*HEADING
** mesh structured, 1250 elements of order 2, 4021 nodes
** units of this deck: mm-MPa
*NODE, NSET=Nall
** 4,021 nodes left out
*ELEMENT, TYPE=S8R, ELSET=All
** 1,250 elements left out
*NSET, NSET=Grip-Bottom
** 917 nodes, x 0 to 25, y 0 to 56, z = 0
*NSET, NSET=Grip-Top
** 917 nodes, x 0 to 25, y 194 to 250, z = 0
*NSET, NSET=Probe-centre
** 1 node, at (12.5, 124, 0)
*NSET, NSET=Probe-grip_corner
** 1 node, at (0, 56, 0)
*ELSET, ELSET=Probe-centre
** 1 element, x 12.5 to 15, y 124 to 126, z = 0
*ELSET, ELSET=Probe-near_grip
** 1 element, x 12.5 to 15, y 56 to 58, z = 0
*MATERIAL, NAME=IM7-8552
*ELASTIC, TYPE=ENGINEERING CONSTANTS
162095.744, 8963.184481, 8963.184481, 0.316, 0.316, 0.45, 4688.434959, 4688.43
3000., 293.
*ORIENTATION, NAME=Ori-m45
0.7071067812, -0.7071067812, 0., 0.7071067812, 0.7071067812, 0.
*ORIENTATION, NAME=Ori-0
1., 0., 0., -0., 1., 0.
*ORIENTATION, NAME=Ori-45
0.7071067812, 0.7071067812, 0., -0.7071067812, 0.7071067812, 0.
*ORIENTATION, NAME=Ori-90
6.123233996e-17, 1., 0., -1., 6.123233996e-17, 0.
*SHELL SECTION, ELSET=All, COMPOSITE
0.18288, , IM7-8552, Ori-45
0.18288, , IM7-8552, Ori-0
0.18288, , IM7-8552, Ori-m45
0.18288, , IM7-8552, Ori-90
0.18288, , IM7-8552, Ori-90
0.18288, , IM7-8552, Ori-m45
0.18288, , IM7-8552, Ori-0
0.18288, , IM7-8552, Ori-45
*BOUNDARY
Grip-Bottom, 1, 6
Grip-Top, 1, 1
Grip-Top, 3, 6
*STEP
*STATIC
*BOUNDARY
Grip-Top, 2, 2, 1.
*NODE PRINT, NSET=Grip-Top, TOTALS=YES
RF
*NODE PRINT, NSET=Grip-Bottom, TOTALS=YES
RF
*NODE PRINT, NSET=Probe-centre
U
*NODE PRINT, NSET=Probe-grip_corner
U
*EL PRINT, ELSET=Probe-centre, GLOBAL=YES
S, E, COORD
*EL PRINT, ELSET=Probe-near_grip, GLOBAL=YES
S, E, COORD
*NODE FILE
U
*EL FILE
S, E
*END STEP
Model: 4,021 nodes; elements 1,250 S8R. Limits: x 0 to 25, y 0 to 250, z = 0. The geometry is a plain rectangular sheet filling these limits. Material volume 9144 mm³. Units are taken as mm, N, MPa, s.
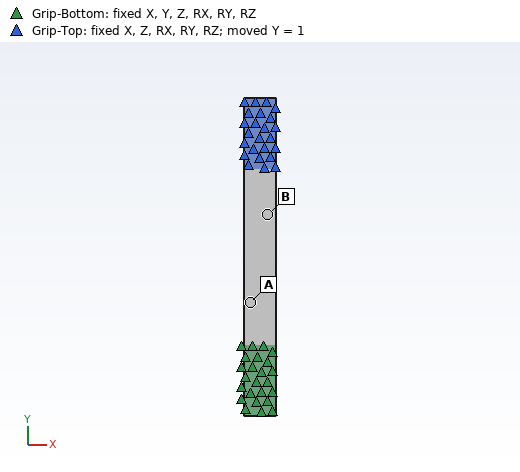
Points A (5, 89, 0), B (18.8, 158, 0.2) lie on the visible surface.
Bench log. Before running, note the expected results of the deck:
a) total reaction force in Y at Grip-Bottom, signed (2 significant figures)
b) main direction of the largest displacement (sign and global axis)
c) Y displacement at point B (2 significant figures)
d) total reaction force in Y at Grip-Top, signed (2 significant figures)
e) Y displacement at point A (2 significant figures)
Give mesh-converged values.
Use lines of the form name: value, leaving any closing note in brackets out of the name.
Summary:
total reaction force in Y at Grip-Bottom, signed: -16000 N
main direction of the largest displacement: +Y
Y displacement at point B: 0.74 mm
total reaction force in Y at Grip-Top, signed: 16000 N
Y displacement at point A: 0.24 mm
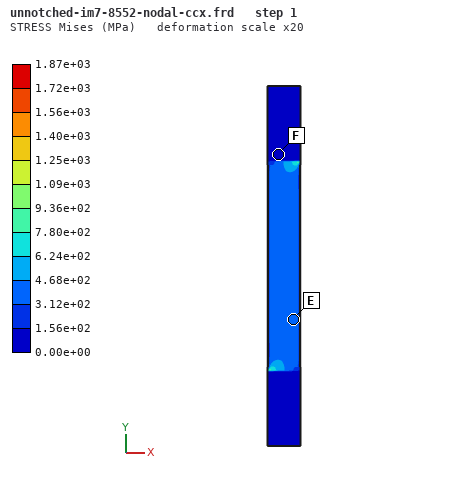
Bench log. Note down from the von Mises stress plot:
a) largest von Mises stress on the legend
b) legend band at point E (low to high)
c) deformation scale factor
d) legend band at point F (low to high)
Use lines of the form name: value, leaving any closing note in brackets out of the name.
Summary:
largest von Mises stress on the legend: 1.87e+03 MPa
legend band at point E: 3.12e+02 to 4.68e+02 MPa
deformation scale factor: 20
legend band at point F: 0.00e+00 to 1.56e+02 MPa
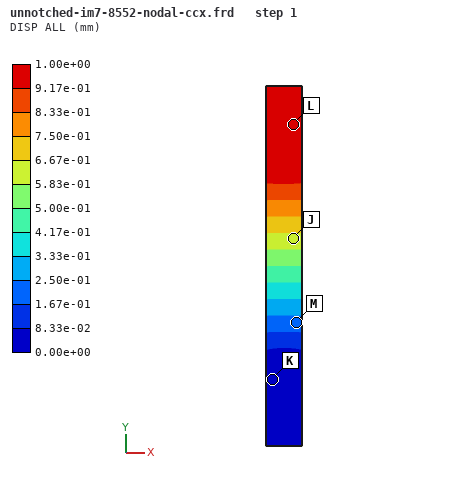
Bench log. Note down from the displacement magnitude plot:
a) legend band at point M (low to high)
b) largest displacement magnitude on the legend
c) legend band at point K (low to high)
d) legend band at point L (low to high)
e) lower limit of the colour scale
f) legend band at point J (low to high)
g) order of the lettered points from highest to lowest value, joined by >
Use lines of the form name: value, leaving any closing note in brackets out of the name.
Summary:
legend band at point M: 1.67e-01 to 2.50e-01 mm
largest displacement magnitude on the legend: 1.00e+00 mm
legend band at point K: 0.00e+00 to 8.33e-02 mm
legend band at point L: 9.17e-01 to 1.00e+00 mm
lower limit of the colour scale: 0.00e+00 mm
legend band at point J: 5.83e-01 to 6.67e-01 mm
order of the lettered points from highest to lowest value, joined by >: L > J > M > K
